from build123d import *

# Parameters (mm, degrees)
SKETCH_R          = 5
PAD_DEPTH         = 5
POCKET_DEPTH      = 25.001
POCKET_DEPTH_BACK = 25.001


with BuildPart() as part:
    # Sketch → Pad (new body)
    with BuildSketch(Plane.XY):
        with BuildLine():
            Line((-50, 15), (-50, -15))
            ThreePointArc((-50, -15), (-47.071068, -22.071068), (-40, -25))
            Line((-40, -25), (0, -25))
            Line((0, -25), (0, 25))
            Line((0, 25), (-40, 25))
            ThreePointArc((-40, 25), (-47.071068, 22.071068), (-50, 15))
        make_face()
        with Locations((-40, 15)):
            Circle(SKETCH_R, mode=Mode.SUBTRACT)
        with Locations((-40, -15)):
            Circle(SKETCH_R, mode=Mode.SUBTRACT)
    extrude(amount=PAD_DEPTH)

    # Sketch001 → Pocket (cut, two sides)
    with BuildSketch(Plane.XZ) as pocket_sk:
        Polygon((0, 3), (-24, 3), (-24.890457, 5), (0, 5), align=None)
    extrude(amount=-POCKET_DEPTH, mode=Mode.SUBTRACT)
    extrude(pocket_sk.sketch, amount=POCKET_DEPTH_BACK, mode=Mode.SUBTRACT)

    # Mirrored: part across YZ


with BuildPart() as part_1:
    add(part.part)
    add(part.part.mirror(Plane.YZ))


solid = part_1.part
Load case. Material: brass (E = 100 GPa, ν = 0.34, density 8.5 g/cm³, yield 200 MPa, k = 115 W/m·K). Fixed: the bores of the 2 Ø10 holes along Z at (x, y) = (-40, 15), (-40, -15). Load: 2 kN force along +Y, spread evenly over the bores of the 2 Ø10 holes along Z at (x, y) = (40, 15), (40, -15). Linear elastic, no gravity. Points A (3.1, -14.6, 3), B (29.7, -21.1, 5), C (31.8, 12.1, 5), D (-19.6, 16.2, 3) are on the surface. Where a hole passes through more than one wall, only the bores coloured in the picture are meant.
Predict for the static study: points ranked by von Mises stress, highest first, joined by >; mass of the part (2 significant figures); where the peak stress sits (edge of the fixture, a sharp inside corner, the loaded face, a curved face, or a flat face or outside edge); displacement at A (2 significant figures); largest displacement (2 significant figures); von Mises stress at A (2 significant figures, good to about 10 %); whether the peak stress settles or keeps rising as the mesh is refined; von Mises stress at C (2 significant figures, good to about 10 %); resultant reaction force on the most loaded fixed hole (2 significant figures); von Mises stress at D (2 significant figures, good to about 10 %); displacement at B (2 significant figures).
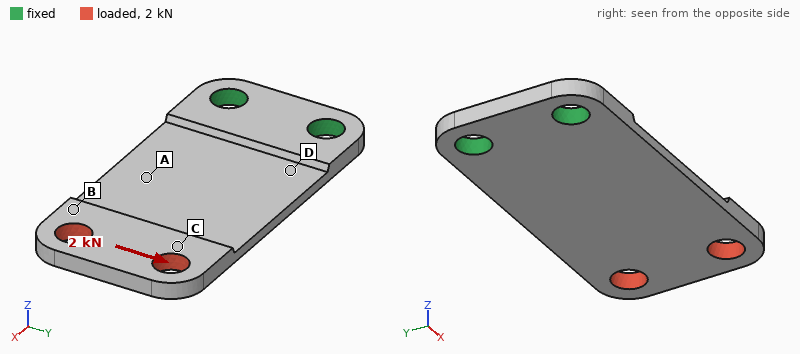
D > A > C > B
150 g
edge of the fixture
0.076 mm
0.20 mm
57 MPa
keeps rising
25 MPa
4.5 kN
74 MPa
0.16 mm
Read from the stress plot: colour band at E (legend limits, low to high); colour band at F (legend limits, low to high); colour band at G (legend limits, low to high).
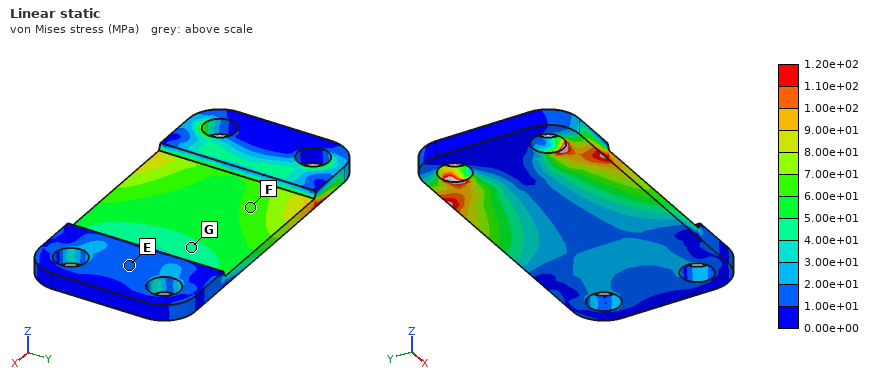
1.00e+01 to 2.00e+01 MPa
6.00e+01 to 7.00e+01 MPa
4.00e+01 to 5.00e+01 MPa
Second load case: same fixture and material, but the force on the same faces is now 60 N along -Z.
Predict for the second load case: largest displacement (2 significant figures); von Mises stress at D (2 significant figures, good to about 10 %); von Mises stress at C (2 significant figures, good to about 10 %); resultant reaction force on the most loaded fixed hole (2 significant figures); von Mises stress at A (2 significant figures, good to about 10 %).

0.64 mm
43 MPa
3.8 MPa
32 N
28 MPa
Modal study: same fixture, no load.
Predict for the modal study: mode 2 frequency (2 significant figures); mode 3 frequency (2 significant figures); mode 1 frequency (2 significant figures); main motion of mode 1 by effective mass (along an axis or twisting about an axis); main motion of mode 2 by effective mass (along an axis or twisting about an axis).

920 Hz
1700 Hz
250 Hz
along Z
twisting about X
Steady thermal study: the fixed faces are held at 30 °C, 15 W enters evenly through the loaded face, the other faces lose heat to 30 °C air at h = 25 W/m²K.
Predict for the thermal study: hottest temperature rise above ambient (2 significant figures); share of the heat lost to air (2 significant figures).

46 K
35 %
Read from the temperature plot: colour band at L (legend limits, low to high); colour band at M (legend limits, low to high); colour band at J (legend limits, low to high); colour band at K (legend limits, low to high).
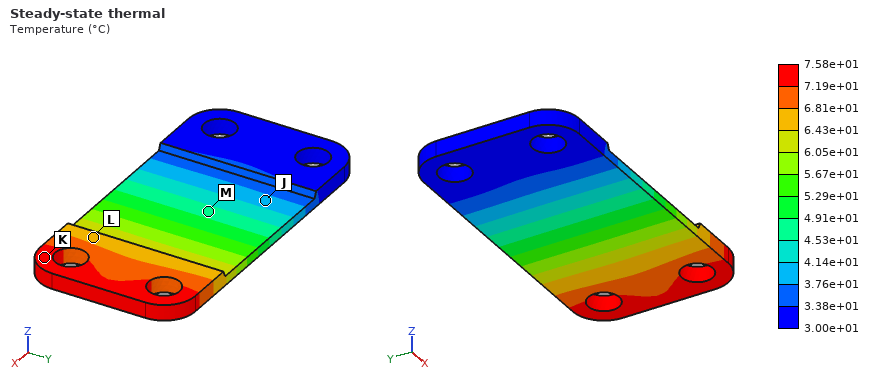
6.43e+01 to 6.81e+01 °C
4.53e+01 to 4.91e+01 °C
3.76e+01 to 4.14e+01 °C
7.19e+01 to 7.58e+01 °C
